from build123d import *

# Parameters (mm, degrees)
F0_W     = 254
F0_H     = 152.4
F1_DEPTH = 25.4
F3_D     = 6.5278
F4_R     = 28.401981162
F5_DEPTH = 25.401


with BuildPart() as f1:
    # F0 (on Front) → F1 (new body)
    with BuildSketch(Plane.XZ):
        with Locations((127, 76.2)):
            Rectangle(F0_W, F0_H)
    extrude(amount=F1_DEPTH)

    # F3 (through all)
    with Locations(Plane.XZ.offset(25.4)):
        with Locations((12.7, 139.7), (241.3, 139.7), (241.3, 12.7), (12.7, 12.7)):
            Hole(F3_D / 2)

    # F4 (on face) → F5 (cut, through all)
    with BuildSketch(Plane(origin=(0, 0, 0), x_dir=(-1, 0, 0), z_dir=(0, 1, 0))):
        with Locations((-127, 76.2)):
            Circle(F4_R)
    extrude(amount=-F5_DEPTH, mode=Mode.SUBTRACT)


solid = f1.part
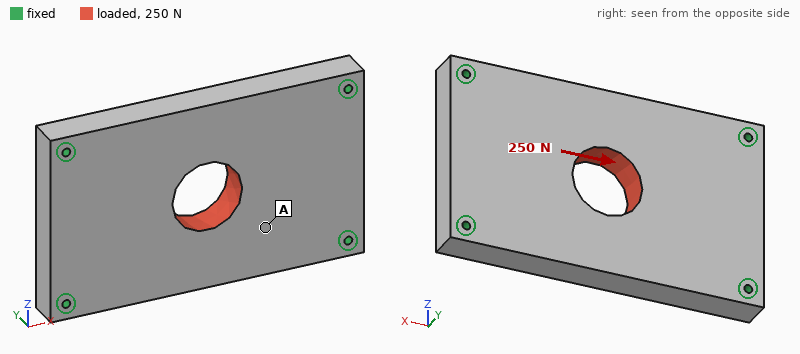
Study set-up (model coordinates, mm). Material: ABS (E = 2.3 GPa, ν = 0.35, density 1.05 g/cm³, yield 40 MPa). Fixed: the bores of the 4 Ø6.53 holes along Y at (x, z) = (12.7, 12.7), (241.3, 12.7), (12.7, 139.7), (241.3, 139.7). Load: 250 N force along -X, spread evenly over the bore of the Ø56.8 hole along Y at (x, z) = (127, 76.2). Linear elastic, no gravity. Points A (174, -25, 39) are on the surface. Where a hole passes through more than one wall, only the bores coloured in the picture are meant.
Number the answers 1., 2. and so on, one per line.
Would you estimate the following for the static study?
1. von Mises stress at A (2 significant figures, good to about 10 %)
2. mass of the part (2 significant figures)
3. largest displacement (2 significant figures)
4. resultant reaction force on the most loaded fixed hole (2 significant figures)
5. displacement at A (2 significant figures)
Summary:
1. 0.044 MPa
2. 960 g
3. 3.0 µm
4. 66 N
5. 2.0 µm
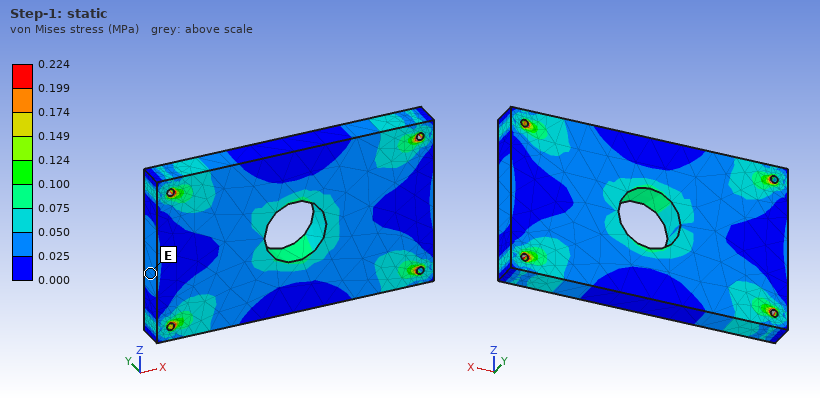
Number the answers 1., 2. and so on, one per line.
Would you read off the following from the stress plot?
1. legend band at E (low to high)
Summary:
1. 0.025 to 0.050 MPa
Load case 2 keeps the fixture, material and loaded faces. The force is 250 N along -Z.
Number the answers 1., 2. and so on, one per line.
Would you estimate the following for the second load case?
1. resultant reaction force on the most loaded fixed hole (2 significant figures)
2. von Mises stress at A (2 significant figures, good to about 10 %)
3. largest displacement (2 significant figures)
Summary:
1. 82 N
2. 0.062 MPa
3. 6.5 µm
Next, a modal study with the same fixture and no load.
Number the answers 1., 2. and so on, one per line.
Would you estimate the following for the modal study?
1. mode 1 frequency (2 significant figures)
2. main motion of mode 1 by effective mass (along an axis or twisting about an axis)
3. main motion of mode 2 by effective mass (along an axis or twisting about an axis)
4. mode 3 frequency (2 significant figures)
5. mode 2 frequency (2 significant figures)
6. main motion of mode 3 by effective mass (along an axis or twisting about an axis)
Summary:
1. 520 Hz
2. along Y
3. twisting about X
4. 1300 Hz
5. 850 Hz
6. twisting about Z
